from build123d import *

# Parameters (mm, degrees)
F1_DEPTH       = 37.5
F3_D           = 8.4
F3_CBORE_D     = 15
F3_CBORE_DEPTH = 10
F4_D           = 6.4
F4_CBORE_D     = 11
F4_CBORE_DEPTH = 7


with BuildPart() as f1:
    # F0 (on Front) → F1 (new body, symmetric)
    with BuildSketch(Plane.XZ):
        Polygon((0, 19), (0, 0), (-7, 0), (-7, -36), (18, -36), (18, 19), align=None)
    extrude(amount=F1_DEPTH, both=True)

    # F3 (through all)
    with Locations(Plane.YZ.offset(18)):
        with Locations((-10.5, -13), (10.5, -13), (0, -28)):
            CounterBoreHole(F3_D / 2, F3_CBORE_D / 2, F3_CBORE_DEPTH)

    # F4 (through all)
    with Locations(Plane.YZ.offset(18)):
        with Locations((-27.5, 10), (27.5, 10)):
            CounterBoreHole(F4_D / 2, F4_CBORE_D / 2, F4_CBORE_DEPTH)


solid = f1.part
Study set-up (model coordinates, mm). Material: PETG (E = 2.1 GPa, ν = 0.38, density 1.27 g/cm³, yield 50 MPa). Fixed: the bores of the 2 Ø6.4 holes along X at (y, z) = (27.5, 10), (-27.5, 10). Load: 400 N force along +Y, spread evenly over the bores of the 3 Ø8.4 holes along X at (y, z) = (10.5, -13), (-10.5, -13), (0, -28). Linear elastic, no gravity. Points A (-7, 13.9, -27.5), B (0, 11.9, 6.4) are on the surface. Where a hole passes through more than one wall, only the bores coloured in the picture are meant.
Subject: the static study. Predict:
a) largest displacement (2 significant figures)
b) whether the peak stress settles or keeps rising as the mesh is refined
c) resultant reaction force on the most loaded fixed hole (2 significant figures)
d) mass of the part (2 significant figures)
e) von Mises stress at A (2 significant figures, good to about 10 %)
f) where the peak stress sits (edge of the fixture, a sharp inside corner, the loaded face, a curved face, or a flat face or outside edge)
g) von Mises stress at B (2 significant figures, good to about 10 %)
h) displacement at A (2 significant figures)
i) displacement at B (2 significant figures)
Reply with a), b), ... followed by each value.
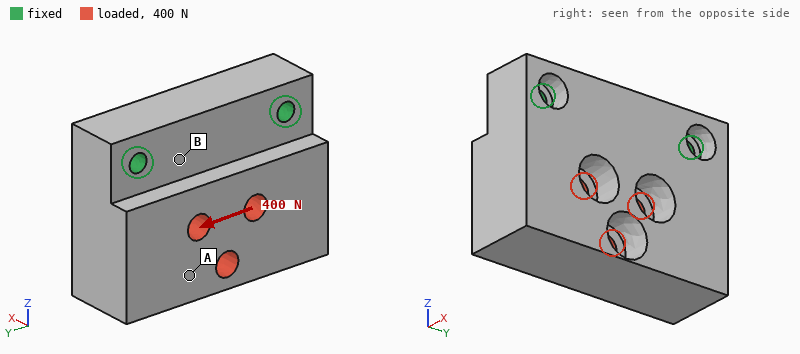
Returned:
a) 34 µm
b) keeps rising
c) 280 N
d) 110 g
e) 0.38 MPa
f) edge of the fixture
g) 0.86 MPa
h) 28 µm
i) 5.6 µm
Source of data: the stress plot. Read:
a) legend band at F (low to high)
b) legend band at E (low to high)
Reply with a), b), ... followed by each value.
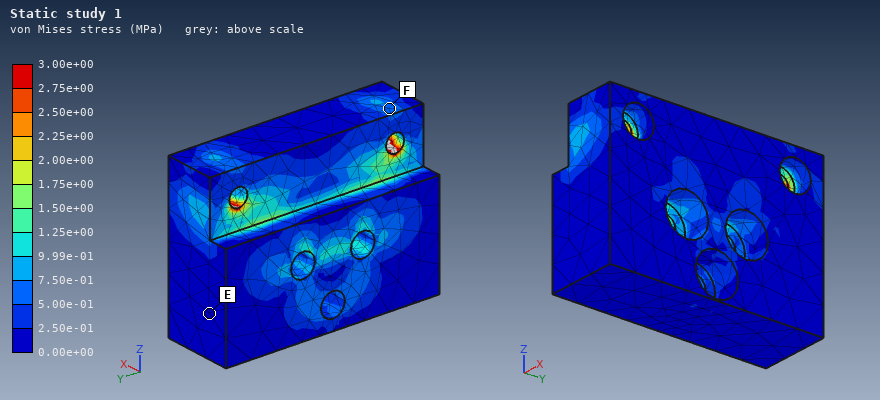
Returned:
a) 5.00e-01 to 7.50e-01 MPa
b) 0.00e+00 to 2.50e-01 MPa
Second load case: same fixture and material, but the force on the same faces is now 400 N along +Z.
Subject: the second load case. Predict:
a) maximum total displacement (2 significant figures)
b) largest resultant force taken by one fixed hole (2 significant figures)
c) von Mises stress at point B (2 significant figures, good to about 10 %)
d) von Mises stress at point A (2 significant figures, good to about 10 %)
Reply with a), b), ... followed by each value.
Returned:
a) 78 µm
b) 210 N
c) 0.84 MPa
d) 0.46 MPa
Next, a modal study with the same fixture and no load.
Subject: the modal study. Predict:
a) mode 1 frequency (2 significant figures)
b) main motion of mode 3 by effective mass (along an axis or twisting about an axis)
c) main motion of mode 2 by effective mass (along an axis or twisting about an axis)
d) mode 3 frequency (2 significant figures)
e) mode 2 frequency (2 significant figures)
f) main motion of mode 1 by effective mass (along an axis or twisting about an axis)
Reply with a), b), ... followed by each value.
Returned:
a) 810 Hz
b) along Y
c) twisting about Z
d) 2400 Hz
e) 1900 Hz
f) along X
